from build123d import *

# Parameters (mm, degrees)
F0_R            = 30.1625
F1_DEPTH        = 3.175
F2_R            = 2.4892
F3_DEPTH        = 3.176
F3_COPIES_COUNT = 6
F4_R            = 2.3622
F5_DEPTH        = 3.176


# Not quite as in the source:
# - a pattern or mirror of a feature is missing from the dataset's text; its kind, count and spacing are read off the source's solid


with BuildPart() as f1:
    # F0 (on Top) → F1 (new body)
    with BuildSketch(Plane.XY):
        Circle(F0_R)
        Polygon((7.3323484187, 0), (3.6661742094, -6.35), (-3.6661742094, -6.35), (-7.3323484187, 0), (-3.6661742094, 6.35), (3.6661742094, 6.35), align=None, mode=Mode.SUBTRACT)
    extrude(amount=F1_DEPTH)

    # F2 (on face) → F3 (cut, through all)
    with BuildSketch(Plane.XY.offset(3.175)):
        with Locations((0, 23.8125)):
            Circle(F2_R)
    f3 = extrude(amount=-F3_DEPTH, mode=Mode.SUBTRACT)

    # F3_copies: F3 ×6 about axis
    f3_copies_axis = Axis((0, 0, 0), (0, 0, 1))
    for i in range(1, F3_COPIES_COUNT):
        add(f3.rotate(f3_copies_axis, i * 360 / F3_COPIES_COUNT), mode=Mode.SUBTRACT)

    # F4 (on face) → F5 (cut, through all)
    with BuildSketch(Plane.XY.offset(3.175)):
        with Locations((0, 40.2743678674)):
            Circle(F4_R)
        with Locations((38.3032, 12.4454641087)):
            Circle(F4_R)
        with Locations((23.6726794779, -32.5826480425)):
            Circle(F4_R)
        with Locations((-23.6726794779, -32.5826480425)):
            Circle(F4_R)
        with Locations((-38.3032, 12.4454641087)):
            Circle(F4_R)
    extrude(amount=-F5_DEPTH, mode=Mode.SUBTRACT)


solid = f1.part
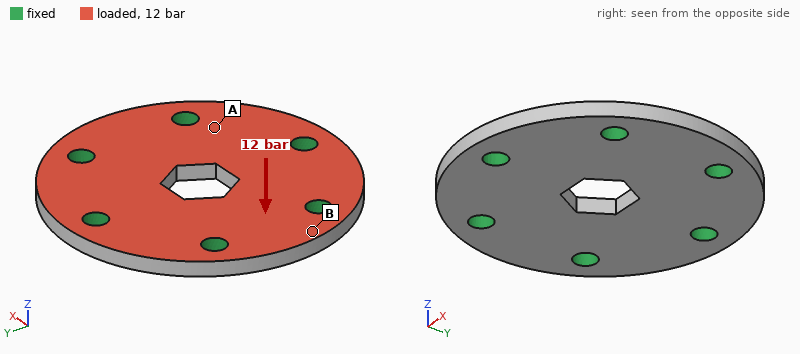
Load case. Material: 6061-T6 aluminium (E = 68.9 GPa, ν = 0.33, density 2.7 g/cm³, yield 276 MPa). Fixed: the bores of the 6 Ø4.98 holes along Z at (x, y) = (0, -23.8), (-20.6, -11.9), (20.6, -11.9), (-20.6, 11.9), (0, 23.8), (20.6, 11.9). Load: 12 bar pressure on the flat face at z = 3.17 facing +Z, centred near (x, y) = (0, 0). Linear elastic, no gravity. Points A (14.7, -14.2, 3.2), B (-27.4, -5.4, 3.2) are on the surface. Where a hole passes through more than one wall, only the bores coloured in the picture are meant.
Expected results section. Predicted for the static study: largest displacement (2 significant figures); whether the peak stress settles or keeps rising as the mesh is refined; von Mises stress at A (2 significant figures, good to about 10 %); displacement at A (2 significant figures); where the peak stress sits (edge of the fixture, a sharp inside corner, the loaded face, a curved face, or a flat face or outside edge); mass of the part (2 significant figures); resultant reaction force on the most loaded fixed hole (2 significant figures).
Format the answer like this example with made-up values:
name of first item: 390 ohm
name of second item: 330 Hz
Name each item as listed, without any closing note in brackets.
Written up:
largest displacement: 27 µm
whether the peak stress settles or keeps rising as the mesh is refined: keeps rising
von Mises stress at A: 22 MPa
displacement at A: 4.1 µm
where the peak stress sits: edge of the fixture
mass of the part: 22 g
resultant reaction force on the most loaded fixed hole: 520 N
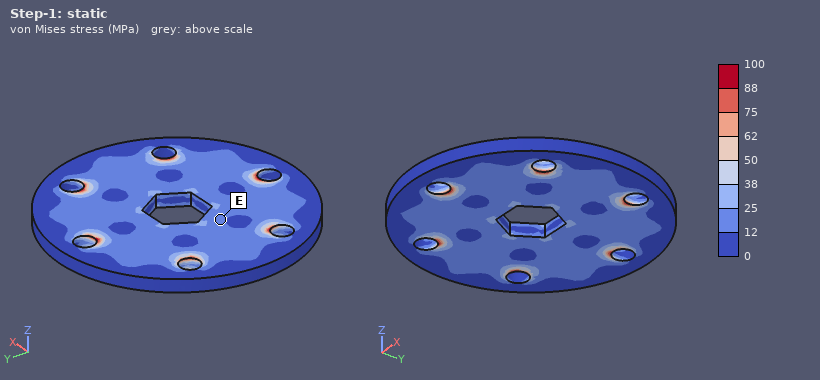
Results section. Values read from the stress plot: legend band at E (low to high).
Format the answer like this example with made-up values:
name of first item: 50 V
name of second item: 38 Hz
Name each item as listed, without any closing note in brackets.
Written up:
legend band at E: 12 to 25 MPa
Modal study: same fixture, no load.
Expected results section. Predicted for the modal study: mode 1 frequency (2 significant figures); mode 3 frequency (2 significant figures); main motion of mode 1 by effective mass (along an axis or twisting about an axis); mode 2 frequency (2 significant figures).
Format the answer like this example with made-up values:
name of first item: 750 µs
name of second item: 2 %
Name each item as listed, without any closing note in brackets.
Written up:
mode 1 frequency: 14 kHz
mode 3 frequency: 23 kHz
main motion of mode 1 by effective mass: along Z
mode 2 frequency: 23 kHz
